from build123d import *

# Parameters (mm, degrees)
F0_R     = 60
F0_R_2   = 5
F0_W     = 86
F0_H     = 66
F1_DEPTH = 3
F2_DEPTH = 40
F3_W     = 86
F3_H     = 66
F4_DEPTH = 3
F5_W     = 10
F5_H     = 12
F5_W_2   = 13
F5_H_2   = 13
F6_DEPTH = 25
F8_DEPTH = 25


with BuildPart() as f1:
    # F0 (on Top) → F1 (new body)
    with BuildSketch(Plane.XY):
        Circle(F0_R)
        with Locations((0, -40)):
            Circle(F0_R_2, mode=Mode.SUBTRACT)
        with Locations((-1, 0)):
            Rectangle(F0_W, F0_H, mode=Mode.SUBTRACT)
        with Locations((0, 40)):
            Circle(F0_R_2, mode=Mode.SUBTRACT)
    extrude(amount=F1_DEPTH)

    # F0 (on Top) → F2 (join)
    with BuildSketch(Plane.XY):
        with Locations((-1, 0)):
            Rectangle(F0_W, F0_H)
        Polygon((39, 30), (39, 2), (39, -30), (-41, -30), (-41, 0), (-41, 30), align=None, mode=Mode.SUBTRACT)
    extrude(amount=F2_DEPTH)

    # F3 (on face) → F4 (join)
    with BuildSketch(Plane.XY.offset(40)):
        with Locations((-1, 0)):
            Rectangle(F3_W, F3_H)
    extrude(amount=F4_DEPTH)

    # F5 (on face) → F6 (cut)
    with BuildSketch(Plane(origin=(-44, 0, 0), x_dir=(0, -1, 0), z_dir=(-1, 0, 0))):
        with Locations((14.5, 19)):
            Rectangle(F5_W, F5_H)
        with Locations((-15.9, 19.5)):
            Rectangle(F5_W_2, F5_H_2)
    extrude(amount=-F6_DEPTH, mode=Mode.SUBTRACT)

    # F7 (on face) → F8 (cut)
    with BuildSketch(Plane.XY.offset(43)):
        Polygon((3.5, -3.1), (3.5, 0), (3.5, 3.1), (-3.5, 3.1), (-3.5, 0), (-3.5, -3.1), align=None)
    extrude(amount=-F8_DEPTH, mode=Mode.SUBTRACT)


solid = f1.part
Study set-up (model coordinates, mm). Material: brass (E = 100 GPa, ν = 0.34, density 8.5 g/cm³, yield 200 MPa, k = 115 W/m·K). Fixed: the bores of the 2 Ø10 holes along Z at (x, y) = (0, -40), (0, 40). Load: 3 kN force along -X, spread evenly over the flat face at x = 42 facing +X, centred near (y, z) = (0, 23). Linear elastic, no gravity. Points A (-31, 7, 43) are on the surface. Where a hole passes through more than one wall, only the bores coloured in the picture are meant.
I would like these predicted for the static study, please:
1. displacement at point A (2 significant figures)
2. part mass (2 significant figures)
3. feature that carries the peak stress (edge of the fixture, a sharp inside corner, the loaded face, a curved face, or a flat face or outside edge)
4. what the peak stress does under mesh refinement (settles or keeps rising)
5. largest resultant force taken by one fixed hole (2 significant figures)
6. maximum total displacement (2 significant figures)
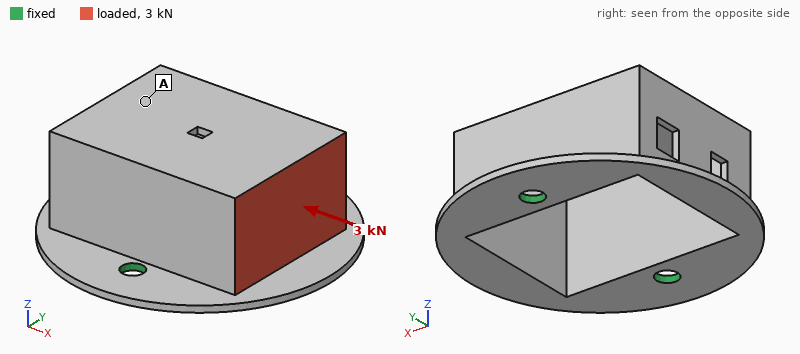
0.34 mm
570 g
edge of the fixture
keeps rising
1.5 kN
0.45 mm
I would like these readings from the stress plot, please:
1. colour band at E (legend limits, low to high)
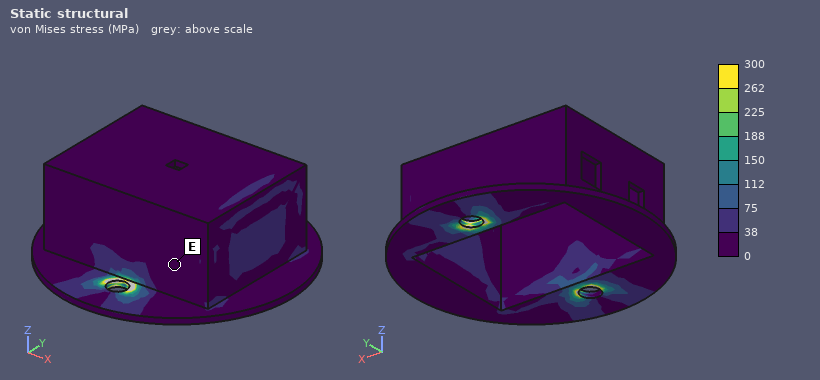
0 to 38 MPa
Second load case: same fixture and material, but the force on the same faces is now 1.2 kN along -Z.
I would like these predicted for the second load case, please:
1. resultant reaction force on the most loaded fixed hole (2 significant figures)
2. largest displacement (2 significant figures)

620 N
0.32 mm
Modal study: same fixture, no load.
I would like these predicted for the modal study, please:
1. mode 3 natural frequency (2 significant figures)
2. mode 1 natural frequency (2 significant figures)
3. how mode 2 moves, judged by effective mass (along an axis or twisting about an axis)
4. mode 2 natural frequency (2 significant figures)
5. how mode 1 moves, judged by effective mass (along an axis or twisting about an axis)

2100 Hz
520 Hz
along Y
2000 Hz
along X
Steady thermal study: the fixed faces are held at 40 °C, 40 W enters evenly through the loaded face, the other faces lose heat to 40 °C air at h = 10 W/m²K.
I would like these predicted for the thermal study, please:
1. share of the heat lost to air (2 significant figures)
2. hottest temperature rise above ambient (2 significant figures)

22 %
48 K
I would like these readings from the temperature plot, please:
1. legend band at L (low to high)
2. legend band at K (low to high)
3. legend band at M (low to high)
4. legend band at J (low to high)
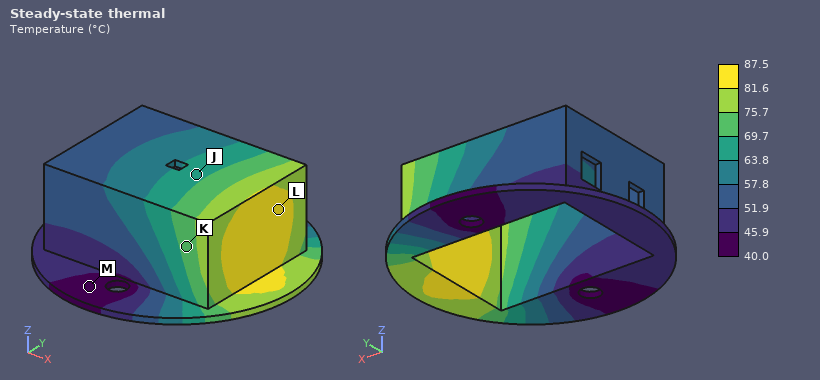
81.6 to 87.5 °C
69.7 to 75.7 °C
40.0 to 45.9 °C
63.8 to 69.7 °C
